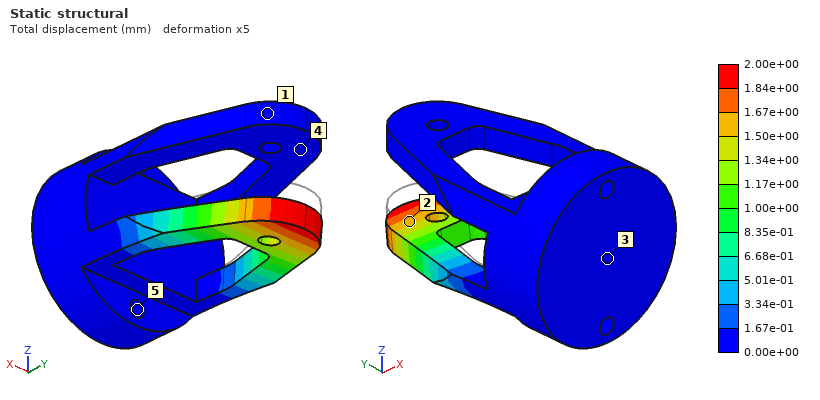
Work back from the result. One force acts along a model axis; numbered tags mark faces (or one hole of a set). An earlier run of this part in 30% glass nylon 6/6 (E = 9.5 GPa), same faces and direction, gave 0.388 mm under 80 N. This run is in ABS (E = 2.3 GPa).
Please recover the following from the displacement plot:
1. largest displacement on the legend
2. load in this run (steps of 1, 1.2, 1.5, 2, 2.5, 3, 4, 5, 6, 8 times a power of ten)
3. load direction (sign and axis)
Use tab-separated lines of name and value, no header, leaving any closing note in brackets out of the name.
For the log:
largest displacement on the legend	2.00e+00 mm
load in this run	100 N
load direction	-Z
